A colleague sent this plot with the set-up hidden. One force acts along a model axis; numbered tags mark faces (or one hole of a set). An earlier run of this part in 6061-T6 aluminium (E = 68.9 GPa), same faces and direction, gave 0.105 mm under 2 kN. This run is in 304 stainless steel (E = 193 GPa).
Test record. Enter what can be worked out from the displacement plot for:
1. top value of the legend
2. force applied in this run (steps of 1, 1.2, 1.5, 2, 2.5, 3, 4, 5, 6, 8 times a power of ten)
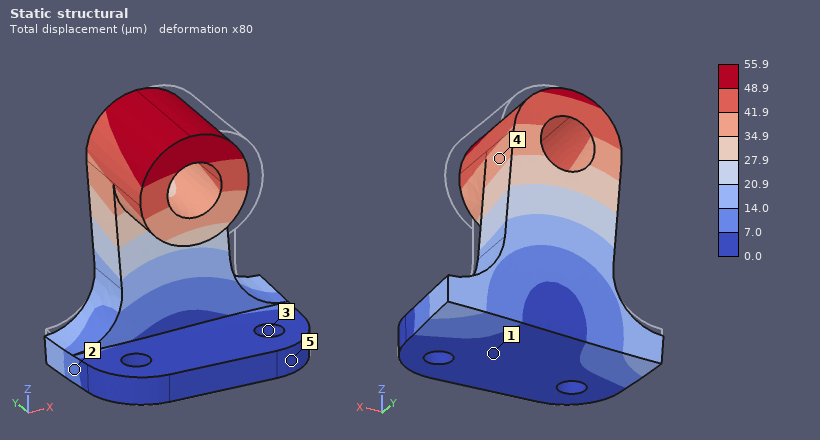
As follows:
55.9 µm
3 kN
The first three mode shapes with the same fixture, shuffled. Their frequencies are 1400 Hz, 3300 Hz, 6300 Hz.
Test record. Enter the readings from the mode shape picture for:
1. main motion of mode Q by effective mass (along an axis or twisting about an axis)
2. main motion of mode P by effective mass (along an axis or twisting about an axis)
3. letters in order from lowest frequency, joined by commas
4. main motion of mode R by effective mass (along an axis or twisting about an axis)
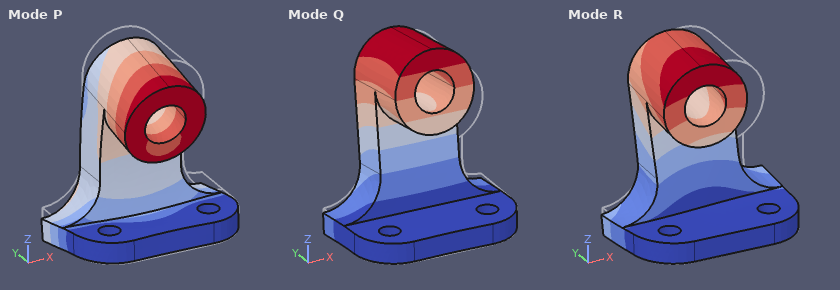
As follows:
along Y
along Z
Q, R, P
along X
